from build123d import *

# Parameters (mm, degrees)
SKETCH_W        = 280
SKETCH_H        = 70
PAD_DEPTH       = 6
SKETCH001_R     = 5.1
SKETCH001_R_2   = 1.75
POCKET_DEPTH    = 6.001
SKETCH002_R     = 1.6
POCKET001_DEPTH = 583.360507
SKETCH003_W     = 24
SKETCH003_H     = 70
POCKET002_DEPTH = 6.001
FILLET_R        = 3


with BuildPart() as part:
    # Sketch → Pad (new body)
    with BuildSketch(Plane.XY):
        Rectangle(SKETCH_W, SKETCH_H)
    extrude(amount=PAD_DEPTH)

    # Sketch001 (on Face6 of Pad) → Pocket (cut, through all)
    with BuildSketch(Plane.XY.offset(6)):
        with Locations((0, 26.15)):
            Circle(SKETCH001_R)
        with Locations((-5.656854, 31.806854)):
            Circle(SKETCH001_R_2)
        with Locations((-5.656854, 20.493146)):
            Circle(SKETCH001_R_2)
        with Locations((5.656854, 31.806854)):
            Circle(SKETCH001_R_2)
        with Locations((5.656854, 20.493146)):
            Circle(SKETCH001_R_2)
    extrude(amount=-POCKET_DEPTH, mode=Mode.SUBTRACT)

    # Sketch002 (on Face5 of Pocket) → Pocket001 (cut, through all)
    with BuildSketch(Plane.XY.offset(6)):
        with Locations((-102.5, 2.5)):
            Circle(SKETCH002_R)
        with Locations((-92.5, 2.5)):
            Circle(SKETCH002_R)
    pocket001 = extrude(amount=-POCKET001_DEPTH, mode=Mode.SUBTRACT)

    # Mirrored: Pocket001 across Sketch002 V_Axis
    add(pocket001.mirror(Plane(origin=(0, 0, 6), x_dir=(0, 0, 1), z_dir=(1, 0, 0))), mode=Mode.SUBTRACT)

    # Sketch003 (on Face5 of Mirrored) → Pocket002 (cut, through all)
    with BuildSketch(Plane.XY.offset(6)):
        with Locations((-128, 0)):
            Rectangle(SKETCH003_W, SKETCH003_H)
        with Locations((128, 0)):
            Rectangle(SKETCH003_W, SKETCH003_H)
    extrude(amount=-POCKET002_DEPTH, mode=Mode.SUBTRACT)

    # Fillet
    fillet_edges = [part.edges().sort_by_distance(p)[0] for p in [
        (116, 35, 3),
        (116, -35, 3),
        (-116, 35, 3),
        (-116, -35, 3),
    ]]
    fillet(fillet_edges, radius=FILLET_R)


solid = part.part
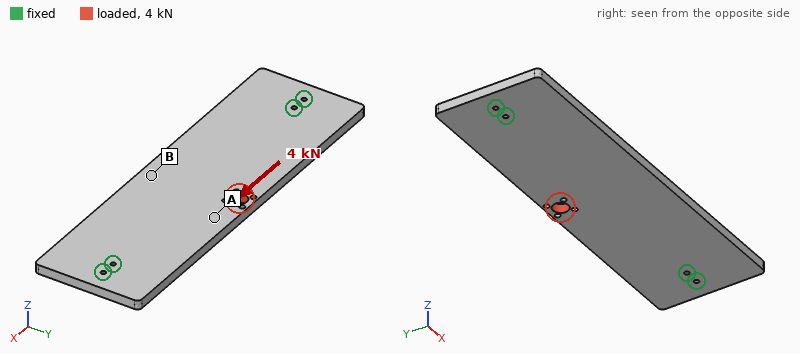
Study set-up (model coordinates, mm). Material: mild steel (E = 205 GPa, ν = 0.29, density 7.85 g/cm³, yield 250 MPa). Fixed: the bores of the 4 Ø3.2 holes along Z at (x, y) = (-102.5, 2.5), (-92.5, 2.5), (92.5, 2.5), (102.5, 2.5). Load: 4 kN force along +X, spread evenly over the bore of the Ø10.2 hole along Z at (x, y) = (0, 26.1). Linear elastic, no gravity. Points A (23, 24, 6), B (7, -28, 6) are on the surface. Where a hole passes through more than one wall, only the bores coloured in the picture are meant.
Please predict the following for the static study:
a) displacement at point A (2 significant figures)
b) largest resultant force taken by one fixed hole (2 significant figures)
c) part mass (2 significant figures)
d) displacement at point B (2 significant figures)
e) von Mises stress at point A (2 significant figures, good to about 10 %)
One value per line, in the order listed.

3.6 µm
1.3 kN
760 g
1.6 µm
12 MPa
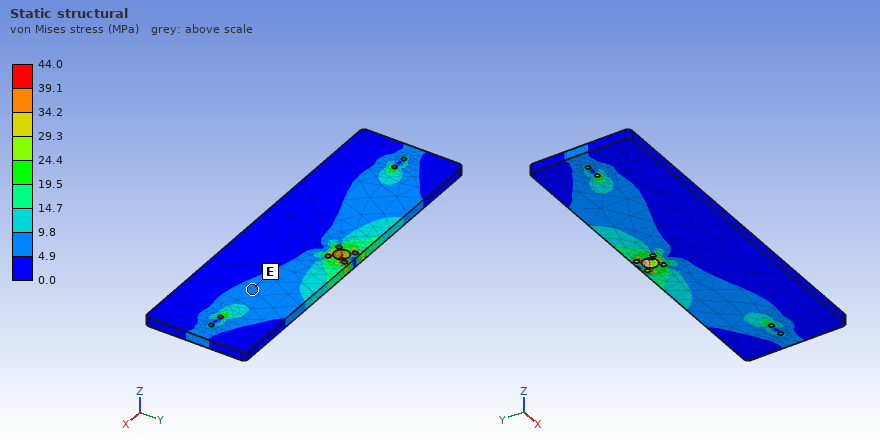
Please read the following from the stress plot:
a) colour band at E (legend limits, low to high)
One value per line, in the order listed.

4.9 to 9.8 MPa
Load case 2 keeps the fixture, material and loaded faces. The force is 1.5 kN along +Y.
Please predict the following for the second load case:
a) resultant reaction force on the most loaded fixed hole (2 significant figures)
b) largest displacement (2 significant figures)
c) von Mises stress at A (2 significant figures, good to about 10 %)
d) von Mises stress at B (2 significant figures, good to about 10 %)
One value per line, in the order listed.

1.3 kN
9.5 µm
5.8 MPa
9.9 MPa
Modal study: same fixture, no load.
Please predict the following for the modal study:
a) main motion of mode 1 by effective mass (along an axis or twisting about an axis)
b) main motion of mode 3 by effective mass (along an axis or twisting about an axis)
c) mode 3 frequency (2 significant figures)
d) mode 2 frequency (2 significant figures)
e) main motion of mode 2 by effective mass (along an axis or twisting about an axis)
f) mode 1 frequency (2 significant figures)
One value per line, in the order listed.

along Z
twisting about Y
2100 Hz
1300 Hz
twisting about X
800 Hz
